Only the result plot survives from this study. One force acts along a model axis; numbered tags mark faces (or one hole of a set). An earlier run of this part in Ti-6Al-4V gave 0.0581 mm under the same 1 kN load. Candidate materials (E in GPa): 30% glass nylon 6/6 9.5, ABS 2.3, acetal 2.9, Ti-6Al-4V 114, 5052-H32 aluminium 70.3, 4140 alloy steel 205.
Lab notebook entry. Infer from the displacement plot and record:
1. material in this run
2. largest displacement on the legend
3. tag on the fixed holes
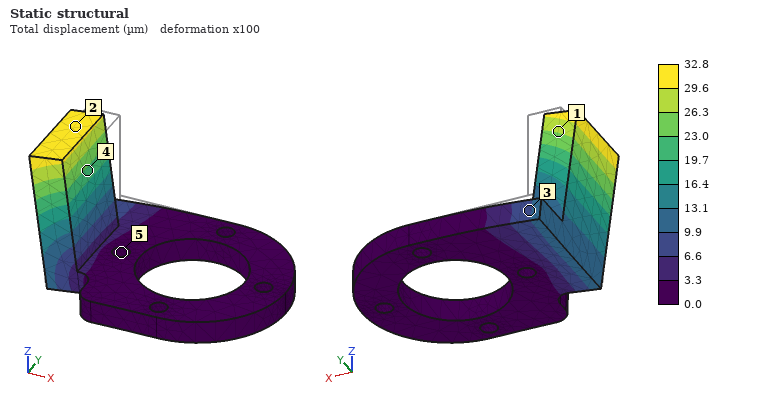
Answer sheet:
4140 alloy steel
32.8 µm
5
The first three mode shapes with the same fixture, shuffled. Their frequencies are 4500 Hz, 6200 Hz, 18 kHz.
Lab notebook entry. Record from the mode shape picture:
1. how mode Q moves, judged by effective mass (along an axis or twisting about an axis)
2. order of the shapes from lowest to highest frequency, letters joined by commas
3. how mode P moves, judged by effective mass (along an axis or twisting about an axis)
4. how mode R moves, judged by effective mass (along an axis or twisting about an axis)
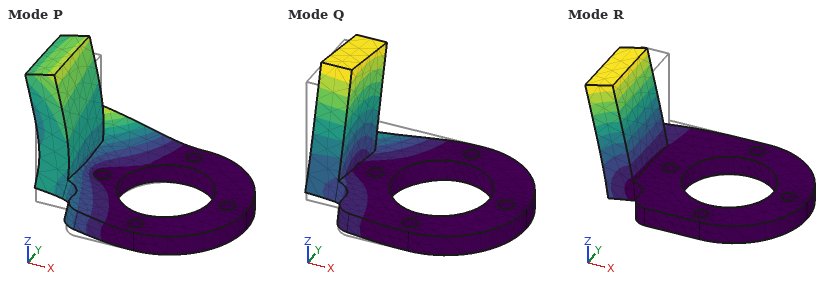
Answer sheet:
along Y
R, Q, P
along Z
along X
